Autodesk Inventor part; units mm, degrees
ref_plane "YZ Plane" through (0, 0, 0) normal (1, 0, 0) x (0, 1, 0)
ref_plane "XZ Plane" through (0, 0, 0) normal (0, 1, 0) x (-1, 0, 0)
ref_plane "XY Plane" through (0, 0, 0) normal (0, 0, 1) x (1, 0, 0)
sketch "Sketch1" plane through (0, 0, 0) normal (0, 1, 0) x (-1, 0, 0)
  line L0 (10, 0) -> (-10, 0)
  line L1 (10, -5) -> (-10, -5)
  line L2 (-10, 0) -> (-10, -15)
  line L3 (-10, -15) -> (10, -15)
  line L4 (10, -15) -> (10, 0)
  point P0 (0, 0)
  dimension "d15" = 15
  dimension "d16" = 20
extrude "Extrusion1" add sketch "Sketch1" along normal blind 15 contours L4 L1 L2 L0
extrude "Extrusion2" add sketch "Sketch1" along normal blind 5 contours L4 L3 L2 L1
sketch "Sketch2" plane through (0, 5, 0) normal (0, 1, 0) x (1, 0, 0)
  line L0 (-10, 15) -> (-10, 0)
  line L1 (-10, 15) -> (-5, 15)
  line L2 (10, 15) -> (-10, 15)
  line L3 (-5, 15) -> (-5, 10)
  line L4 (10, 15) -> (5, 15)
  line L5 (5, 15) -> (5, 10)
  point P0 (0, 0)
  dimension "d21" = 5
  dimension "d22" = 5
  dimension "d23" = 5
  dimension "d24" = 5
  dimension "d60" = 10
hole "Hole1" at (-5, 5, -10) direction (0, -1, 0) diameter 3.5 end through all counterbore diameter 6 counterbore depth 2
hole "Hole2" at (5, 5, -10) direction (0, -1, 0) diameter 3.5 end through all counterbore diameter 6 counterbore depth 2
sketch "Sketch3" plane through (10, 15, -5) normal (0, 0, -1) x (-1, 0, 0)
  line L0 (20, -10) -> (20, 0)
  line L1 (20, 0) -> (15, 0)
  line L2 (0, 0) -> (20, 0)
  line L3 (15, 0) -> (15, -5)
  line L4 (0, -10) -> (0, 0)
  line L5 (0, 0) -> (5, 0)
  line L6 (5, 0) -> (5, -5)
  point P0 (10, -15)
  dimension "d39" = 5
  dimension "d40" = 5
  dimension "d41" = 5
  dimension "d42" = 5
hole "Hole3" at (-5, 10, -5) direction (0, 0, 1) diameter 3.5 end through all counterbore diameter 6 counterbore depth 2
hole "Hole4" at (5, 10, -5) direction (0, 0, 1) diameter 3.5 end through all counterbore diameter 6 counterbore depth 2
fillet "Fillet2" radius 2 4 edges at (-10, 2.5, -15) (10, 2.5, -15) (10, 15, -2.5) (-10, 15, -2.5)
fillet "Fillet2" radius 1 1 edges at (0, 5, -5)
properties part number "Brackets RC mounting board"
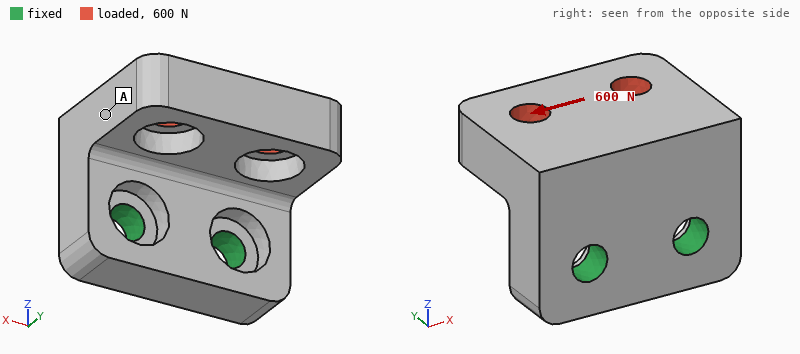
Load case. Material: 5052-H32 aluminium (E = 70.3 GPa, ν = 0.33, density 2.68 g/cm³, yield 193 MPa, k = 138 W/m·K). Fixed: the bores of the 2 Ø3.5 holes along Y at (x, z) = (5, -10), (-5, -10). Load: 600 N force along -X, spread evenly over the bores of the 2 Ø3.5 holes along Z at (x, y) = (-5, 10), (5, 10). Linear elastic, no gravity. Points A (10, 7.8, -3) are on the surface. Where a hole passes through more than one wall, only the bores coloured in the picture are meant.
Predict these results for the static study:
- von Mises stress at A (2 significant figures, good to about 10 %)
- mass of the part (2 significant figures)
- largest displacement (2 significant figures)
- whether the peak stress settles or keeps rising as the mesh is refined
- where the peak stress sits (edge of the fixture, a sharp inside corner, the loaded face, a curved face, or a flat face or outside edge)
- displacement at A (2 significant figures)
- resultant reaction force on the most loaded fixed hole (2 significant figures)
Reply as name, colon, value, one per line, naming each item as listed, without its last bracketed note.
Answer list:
von Mises stress at A: 11 MPa
mass of the part: 5.7 g
largest displacement: 18 µm
whether the peak stress settles or keeps rising as the mesh is refined: keeps rising
where the peak stress sits: edge of the fixture
displacement at A: 12 µm
resultant reaction force on the most loaded fixed hole: 640 N
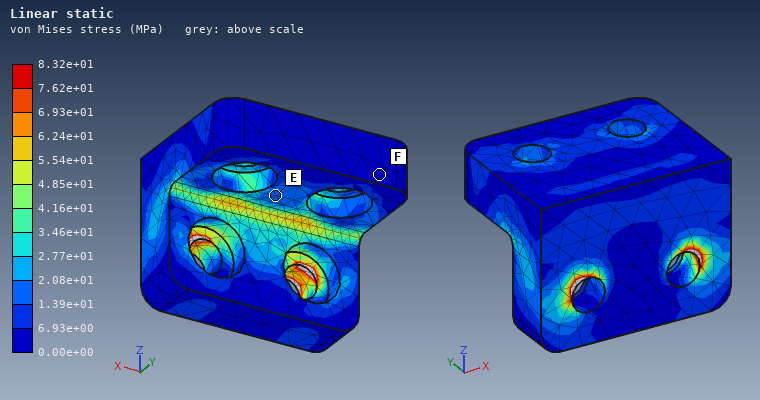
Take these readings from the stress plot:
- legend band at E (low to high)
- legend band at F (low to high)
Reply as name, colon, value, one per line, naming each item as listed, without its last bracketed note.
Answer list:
legend band at E: 1.39e+01 to 2.08e+01 MPa
legend band at F: 0.00e+00 to 6.93e+00 MPa
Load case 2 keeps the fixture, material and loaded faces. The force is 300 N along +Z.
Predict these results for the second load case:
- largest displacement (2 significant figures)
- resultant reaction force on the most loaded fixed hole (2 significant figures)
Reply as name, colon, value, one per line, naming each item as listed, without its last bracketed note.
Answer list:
largest displacement: 30 µm
resultant reaction force on the most loaded fixed hole: 150 N
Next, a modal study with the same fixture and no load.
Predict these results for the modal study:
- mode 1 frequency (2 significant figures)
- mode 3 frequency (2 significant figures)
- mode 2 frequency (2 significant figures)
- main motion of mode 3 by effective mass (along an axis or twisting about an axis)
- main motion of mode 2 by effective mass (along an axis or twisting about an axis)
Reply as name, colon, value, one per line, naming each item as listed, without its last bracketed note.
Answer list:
mode 1 frequency: 11 kHz
mode 3 frequency: 30 kHz
mode 2 frequency: 19 kHz
main motion of mode 3 by effective mass: along X
main motion of mode 2 by effective mass: along X
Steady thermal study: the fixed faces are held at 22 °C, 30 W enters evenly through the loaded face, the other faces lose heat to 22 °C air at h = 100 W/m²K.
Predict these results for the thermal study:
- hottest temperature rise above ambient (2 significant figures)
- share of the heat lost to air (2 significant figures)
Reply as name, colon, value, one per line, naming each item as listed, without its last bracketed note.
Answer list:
hottest temperature rise above ambient: 36 K
share of the heat lost to air: 7.7 %
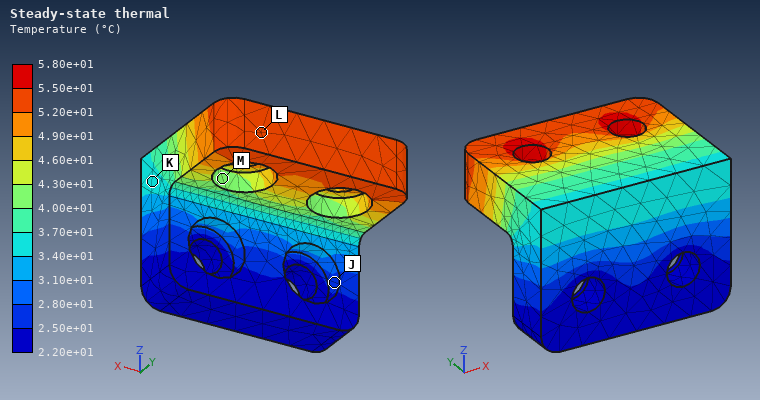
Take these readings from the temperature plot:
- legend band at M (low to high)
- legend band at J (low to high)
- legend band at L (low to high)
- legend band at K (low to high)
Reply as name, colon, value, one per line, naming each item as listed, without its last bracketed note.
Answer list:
legend band at M: 4.00e+01 to 4.30e+01 °C
legend band at J: 2.50e+01 to 2.80e+01 °C
legend band at L: 5.20e+01 to 5.50e+01 °C
legend band at K: 3.40e+01 to 3.70e+01 °C
